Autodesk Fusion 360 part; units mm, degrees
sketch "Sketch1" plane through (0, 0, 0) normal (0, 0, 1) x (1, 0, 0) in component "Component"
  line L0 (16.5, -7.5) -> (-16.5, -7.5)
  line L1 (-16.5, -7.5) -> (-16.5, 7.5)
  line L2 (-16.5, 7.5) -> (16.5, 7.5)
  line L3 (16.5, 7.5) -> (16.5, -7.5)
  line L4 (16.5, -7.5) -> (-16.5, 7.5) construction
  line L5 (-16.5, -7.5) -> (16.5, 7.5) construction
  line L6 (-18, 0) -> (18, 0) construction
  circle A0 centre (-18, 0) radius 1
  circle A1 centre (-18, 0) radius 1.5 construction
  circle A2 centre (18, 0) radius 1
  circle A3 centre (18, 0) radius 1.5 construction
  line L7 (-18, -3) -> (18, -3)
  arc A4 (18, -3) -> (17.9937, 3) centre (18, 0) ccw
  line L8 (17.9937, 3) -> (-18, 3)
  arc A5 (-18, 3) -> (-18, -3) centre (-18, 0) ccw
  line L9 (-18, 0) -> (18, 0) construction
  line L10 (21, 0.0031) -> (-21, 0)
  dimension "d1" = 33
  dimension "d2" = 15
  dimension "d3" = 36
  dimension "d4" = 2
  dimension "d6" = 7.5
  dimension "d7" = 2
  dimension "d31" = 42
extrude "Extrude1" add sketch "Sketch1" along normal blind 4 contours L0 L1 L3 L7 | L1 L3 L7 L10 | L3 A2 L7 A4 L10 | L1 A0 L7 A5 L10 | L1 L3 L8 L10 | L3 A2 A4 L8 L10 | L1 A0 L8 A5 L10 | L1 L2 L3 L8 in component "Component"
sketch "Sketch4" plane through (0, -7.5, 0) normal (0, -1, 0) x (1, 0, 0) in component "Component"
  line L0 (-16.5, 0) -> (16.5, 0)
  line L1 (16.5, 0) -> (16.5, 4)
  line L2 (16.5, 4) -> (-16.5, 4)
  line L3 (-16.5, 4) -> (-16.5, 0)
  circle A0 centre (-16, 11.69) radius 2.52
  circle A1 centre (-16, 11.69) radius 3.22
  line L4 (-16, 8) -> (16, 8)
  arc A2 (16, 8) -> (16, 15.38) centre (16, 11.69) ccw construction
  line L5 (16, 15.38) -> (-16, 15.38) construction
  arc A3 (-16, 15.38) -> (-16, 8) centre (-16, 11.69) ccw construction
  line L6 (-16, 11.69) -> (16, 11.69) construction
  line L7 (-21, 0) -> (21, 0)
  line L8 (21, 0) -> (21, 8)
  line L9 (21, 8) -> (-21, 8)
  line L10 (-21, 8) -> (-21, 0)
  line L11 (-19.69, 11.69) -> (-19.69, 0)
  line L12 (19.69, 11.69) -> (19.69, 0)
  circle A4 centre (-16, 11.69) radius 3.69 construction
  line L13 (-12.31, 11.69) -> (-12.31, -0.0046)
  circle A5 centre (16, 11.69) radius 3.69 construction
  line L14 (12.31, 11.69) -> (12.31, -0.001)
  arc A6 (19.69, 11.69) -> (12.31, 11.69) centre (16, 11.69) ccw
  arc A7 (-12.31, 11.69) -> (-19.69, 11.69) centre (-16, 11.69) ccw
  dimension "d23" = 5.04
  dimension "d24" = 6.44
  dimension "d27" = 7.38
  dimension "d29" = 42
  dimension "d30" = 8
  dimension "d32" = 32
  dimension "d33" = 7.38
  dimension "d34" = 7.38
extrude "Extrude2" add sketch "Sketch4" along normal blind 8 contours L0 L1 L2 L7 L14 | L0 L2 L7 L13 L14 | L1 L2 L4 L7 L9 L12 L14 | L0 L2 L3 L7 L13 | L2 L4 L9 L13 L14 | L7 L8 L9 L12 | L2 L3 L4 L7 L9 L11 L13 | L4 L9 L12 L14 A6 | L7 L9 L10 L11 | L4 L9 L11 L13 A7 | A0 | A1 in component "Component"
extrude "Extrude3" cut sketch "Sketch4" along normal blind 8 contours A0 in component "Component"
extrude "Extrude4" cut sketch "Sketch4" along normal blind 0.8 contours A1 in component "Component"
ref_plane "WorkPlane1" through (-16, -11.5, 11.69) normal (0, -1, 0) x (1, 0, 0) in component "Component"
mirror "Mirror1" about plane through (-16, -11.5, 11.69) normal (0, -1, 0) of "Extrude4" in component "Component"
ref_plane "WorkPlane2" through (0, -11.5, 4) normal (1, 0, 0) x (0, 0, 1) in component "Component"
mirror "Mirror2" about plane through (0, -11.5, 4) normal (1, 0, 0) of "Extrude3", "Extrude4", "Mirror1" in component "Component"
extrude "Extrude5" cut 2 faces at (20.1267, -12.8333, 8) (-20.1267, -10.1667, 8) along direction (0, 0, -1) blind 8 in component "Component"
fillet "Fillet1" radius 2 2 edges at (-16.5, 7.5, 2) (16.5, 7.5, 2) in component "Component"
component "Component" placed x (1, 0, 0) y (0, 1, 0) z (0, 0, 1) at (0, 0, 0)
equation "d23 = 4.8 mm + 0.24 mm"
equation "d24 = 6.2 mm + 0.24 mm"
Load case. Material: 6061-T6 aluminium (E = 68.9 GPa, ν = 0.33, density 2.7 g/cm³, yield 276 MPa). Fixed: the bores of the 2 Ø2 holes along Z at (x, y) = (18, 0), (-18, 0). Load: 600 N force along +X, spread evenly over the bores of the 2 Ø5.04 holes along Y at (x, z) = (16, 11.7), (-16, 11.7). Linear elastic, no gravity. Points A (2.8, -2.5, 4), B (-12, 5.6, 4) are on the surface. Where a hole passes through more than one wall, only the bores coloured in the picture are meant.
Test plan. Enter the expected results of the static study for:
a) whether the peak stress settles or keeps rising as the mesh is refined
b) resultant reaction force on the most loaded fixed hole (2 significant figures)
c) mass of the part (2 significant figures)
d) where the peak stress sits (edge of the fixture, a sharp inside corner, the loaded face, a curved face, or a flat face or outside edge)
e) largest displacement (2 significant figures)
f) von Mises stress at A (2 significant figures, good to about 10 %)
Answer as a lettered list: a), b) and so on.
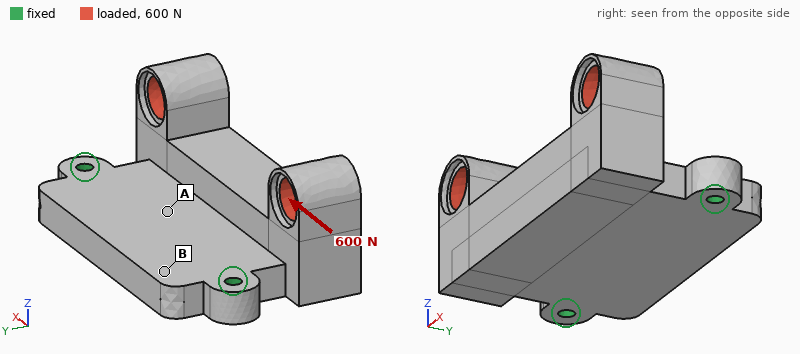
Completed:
a) keeps rising
b) 400 N
c) 14 g
d) edge of the fixture
e) 40 µm
f) 15 MPa
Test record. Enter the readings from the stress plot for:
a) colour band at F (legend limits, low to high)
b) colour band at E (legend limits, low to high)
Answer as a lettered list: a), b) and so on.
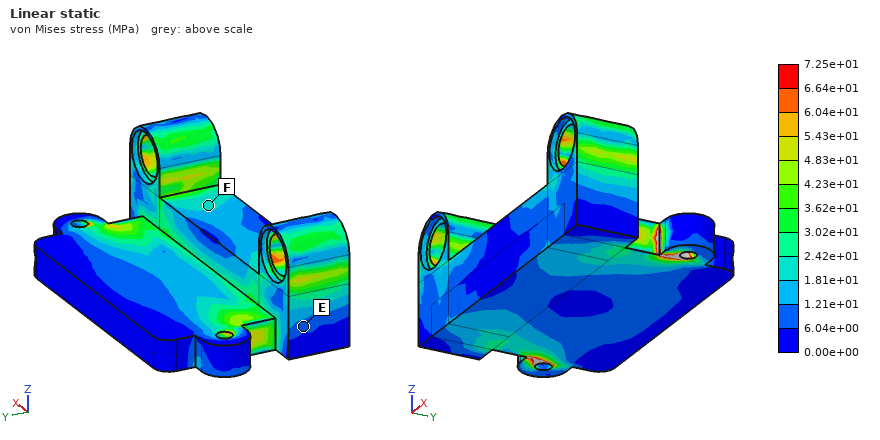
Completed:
a) 1.81e+01 to 2.42e+01 MPa
b) 6.04e+00 to 1.21e+01 MPa
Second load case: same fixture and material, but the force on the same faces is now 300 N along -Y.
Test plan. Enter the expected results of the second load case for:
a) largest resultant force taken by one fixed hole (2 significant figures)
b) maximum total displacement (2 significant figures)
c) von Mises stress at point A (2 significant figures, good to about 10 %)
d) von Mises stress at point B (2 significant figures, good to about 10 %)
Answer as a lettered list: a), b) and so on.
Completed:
a) 150 N
b) 88 µm
c) 16 MPa
d) 13 MPa
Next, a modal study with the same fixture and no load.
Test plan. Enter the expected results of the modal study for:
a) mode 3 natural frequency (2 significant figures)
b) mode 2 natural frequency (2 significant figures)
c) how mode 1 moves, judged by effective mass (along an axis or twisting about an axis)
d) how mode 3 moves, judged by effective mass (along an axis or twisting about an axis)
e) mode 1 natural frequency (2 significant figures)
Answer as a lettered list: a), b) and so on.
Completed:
a) 13 kHz
b) 9700 Hz
c) along Z
d) along Z
e) 4200 Hz
